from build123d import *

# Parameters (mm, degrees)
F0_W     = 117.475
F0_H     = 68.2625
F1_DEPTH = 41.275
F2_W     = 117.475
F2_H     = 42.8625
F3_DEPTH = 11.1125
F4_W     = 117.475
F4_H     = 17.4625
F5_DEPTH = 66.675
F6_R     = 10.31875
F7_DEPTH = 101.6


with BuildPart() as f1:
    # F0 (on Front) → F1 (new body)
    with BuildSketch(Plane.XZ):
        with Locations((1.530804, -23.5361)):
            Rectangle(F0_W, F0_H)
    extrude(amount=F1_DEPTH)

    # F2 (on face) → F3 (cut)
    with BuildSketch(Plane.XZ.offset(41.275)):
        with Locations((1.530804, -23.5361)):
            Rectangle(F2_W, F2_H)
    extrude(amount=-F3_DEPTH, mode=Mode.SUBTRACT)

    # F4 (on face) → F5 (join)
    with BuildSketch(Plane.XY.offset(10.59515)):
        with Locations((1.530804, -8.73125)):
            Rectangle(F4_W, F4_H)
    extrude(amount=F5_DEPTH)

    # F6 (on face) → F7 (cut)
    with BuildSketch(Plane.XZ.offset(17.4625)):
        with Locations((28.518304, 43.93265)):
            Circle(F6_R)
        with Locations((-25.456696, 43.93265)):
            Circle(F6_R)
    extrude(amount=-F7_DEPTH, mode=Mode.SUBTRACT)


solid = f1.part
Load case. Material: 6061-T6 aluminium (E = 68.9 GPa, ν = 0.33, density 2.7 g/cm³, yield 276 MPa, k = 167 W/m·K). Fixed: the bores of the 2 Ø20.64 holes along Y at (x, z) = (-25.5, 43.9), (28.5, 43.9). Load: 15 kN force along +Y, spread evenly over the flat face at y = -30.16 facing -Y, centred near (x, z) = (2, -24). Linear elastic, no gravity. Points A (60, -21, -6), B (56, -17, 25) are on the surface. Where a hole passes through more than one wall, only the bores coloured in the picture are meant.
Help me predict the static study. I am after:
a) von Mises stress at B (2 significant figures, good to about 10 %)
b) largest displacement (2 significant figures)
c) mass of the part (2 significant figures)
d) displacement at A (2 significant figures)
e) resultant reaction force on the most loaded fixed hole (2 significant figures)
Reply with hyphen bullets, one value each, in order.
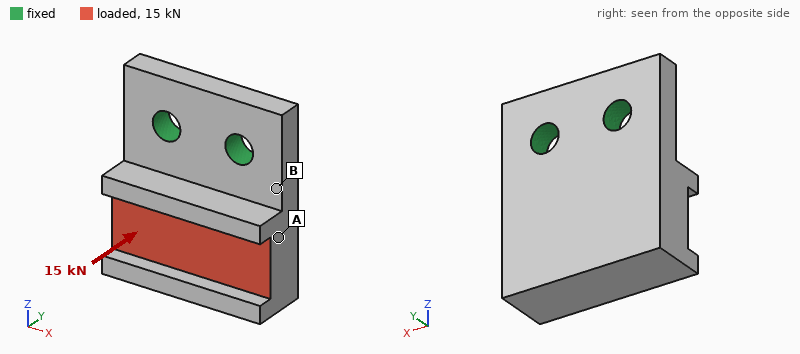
- 90 MPa
- 0.59 mm
- 1.1 kg
- 0.22 mm
- 7.5 kN
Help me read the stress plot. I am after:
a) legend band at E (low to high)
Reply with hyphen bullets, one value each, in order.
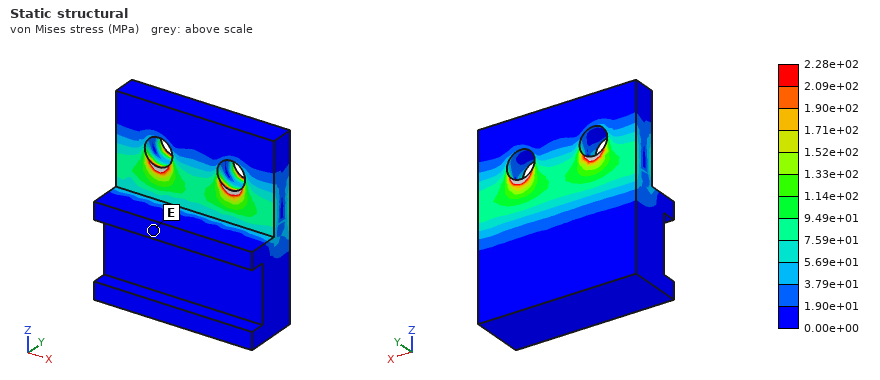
- 0.00e+00 to 1.90e+01 MPa
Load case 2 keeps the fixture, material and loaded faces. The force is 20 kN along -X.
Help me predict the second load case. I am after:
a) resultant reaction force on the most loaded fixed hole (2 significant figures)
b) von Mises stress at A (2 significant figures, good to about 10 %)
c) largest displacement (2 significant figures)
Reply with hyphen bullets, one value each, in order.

- 21 kN
- 15 MPa
- 0.11 mm
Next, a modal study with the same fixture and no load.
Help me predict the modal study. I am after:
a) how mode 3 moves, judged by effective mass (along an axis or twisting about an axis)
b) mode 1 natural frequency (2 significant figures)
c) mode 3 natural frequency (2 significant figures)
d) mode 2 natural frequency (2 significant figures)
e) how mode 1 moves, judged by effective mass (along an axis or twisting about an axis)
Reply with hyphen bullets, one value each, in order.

- along X
- 1100 Hz
- 3800 Hz
- 2900 Hz
- along Y
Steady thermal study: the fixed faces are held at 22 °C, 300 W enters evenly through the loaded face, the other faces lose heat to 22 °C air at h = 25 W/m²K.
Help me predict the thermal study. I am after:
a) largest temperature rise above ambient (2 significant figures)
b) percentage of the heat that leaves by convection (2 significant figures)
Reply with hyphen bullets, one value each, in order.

- 45 K
- 9.1 %
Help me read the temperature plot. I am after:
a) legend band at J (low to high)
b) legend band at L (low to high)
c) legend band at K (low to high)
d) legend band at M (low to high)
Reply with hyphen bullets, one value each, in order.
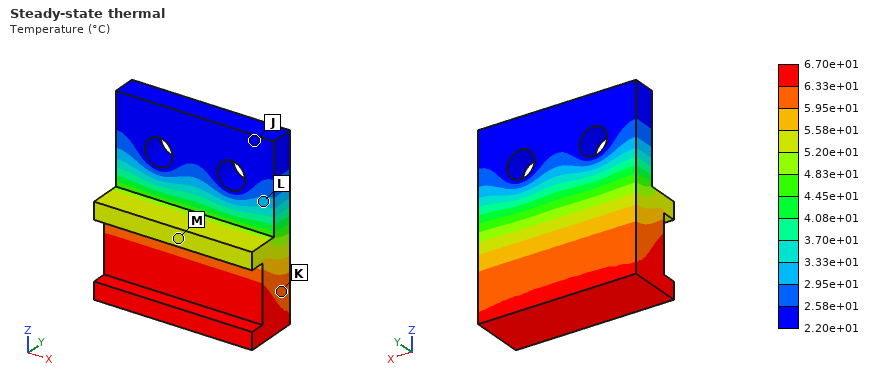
- 2.20e+01 to 2.58e+01 °C
- 2.95e+01 to 3.33e+01 °C
- 5.95e+01 to 6.33e+01 °C
- 5.20e+01 to 5.58e+01 °C
